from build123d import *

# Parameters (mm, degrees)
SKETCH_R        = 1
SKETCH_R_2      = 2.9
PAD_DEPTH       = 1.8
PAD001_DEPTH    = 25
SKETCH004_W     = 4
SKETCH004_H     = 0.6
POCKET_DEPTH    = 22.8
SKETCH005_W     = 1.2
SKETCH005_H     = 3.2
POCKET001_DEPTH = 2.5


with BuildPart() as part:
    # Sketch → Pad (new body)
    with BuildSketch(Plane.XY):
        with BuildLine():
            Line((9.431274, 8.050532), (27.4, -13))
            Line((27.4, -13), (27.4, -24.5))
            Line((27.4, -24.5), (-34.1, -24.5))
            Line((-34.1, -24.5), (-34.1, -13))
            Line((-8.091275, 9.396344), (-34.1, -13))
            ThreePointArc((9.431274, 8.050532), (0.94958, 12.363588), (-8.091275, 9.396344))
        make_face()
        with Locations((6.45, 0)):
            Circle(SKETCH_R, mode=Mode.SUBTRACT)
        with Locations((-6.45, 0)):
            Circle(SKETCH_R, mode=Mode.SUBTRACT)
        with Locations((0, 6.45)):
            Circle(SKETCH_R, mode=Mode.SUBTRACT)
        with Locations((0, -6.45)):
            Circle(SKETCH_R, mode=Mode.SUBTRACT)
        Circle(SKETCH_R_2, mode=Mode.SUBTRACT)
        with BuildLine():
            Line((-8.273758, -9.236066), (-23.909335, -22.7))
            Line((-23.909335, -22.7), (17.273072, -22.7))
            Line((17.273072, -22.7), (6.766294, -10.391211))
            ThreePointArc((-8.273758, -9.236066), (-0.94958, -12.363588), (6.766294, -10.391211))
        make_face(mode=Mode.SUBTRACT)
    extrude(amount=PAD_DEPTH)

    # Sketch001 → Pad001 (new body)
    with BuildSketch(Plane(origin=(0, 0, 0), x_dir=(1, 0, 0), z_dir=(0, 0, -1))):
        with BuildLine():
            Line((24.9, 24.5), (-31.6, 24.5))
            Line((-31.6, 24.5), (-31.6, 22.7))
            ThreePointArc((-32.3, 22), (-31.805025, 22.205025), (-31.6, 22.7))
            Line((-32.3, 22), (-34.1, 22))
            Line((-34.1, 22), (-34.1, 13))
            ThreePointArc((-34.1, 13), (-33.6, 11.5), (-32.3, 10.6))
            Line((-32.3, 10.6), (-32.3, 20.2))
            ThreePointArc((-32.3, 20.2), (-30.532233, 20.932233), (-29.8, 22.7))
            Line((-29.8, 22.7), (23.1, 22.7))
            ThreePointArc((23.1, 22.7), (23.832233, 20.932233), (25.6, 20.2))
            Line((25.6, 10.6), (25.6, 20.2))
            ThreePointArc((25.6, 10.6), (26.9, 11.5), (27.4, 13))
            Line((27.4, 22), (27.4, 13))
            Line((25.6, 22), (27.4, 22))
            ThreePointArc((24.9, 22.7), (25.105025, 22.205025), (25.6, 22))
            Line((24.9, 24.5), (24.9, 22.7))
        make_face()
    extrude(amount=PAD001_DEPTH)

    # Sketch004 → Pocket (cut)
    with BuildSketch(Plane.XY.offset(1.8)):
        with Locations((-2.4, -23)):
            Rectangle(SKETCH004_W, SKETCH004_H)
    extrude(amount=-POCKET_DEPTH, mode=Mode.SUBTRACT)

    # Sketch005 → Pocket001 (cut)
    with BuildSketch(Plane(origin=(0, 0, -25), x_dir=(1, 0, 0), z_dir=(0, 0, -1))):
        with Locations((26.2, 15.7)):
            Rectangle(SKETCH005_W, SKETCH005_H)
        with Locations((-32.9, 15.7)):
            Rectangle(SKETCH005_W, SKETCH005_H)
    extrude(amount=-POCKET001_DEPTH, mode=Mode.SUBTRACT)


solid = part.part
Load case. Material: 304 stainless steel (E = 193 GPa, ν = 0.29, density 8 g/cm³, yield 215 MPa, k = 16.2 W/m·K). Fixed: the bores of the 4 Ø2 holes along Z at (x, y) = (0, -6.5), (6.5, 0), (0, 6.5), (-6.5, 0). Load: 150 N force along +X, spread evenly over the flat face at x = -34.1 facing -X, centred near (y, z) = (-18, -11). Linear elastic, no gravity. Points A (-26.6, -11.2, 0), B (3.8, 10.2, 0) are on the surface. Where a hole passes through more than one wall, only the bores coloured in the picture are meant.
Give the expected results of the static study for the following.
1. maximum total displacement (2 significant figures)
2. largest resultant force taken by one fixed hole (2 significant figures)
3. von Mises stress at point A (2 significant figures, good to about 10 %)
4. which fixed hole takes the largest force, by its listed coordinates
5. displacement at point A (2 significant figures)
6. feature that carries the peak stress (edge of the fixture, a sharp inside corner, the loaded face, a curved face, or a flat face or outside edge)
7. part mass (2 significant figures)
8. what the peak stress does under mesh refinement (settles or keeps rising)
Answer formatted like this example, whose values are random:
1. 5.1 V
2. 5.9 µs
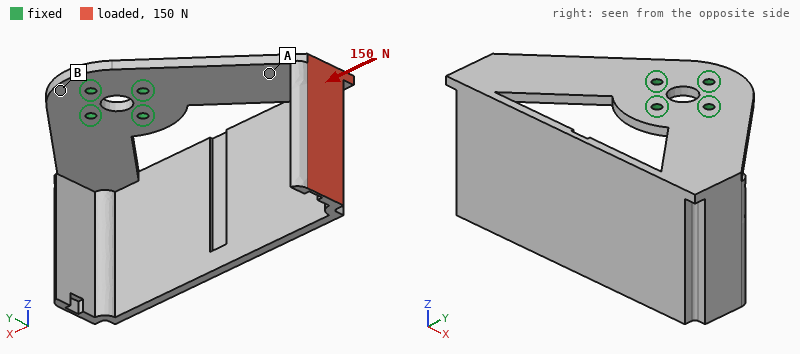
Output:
1. 0.26 mm
2. 210 N
3. 25 MPa
4. (0, -6.5)
5. 0.11 mm
6. edge of the fixture
7. 47 g
8. keeps rising
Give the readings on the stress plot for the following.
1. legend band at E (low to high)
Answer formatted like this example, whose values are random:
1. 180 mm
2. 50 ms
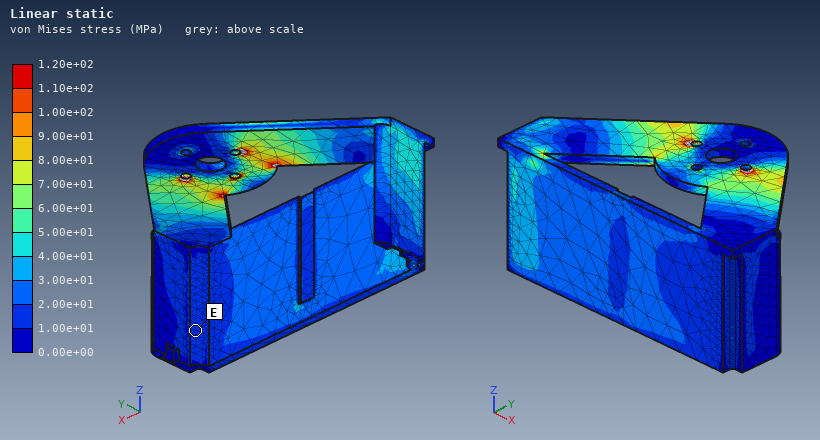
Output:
1. 1.00e+01 to 2.00e+01 MPa
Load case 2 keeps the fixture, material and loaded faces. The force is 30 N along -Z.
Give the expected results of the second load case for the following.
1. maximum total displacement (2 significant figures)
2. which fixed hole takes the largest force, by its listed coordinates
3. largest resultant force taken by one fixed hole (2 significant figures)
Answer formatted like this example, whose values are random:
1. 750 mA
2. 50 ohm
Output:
1. 0.16 mm
2. (-6.5, 0)
3. 53 N
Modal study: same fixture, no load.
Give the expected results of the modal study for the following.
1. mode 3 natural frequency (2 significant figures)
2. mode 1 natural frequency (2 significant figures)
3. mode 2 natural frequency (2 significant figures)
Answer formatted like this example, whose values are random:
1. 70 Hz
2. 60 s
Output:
1. 1300 Hz
2. 530 Hz
3. 640 Hz
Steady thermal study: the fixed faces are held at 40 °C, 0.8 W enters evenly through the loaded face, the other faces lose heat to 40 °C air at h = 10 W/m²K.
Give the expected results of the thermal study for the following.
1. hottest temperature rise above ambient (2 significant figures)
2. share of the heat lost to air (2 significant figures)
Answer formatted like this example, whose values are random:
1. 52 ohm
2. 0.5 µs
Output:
1. 25 K
2. 69 %
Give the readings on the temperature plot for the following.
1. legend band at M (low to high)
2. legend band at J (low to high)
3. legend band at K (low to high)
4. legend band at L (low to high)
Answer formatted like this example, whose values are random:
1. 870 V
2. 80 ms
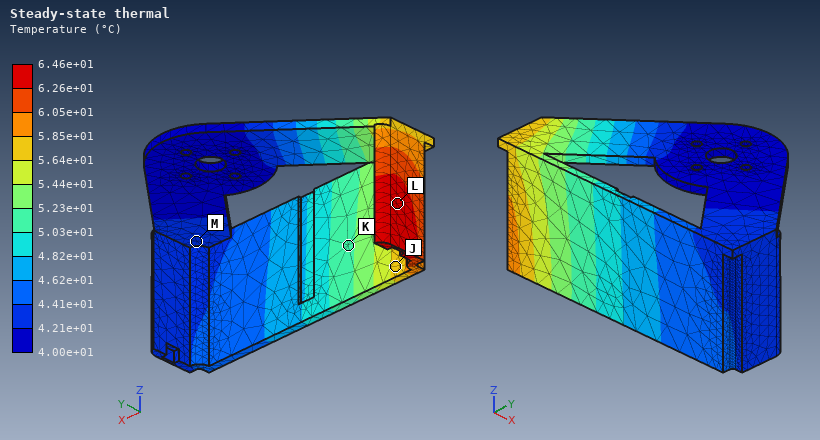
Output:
1. 4.21e+01 to 4.41e+01 °C
2. 5.64e+01 to 5.85e+01 °C
3. 5.03e+01 to 5.23e+01 °C
4. 6.26e+01 to 6.46e+01 °C
